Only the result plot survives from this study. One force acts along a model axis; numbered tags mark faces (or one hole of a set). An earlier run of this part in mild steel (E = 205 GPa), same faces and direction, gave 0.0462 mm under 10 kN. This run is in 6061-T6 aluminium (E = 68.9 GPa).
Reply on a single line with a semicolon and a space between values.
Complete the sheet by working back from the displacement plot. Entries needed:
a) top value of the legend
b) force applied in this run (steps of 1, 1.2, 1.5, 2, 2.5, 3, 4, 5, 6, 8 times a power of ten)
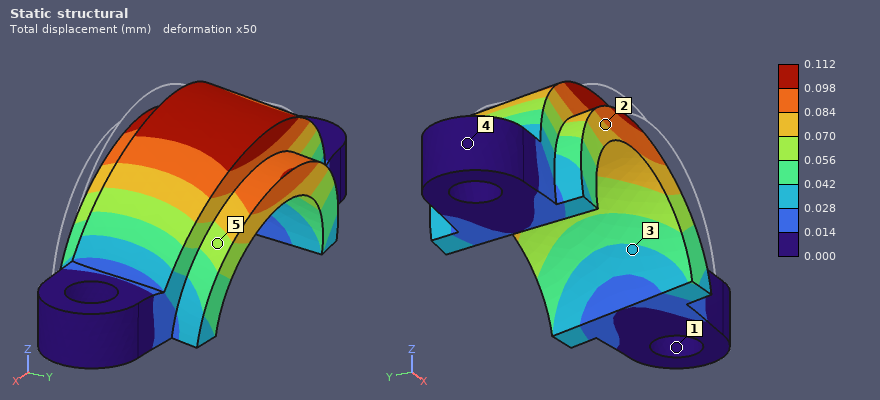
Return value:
0.112 mm; 8 kN
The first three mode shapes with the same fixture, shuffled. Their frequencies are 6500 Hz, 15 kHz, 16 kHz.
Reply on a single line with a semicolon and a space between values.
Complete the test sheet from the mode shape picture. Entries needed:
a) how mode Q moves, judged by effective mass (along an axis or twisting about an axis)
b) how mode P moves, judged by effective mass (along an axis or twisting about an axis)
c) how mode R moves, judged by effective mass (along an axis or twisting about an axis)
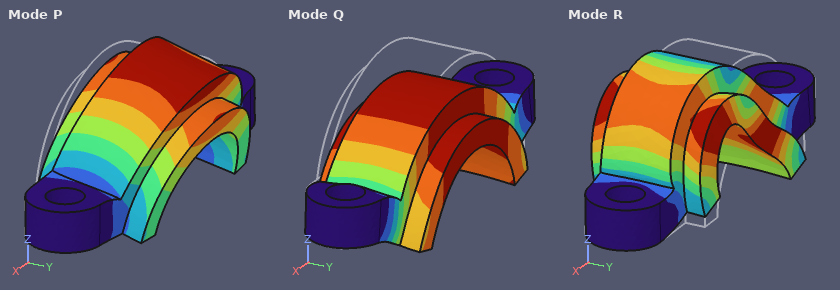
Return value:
along Z; along Y; along X
